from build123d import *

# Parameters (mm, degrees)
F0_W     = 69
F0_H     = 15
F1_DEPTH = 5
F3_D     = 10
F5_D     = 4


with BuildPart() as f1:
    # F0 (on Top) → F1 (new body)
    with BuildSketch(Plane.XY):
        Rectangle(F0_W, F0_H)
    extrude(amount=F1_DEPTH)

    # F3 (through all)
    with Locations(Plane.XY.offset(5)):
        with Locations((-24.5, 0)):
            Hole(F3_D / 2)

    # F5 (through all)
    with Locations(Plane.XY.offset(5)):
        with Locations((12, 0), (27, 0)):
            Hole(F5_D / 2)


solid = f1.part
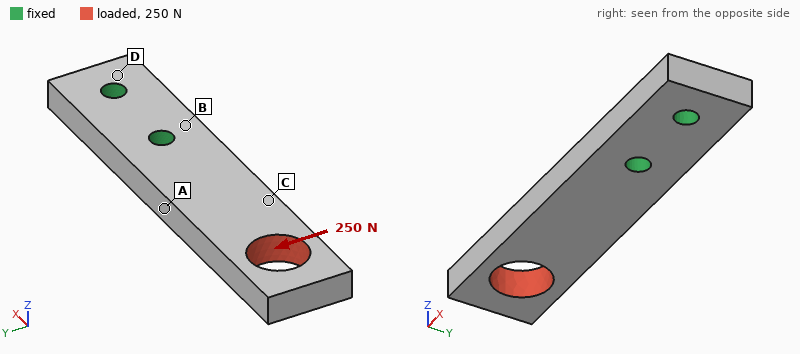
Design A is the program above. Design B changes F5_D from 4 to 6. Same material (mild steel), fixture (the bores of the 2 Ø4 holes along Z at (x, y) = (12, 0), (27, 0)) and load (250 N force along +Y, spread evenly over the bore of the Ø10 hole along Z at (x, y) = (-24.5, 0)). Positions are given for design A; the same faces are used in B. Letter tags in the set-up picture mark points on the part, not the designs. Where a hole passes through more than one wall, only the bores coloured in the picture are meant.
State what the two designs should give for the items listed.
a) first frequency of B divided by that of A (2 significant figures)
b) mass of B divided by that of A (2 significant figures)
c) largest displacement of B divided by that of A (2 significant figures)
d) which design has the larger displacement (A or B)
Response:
1.1
0.97
0.87
A
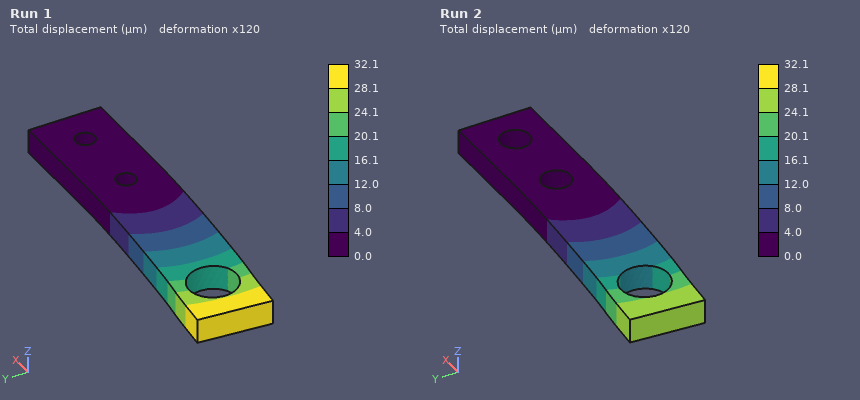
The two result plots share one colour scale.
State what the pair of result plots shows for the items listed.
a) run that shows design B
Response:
Run 2
